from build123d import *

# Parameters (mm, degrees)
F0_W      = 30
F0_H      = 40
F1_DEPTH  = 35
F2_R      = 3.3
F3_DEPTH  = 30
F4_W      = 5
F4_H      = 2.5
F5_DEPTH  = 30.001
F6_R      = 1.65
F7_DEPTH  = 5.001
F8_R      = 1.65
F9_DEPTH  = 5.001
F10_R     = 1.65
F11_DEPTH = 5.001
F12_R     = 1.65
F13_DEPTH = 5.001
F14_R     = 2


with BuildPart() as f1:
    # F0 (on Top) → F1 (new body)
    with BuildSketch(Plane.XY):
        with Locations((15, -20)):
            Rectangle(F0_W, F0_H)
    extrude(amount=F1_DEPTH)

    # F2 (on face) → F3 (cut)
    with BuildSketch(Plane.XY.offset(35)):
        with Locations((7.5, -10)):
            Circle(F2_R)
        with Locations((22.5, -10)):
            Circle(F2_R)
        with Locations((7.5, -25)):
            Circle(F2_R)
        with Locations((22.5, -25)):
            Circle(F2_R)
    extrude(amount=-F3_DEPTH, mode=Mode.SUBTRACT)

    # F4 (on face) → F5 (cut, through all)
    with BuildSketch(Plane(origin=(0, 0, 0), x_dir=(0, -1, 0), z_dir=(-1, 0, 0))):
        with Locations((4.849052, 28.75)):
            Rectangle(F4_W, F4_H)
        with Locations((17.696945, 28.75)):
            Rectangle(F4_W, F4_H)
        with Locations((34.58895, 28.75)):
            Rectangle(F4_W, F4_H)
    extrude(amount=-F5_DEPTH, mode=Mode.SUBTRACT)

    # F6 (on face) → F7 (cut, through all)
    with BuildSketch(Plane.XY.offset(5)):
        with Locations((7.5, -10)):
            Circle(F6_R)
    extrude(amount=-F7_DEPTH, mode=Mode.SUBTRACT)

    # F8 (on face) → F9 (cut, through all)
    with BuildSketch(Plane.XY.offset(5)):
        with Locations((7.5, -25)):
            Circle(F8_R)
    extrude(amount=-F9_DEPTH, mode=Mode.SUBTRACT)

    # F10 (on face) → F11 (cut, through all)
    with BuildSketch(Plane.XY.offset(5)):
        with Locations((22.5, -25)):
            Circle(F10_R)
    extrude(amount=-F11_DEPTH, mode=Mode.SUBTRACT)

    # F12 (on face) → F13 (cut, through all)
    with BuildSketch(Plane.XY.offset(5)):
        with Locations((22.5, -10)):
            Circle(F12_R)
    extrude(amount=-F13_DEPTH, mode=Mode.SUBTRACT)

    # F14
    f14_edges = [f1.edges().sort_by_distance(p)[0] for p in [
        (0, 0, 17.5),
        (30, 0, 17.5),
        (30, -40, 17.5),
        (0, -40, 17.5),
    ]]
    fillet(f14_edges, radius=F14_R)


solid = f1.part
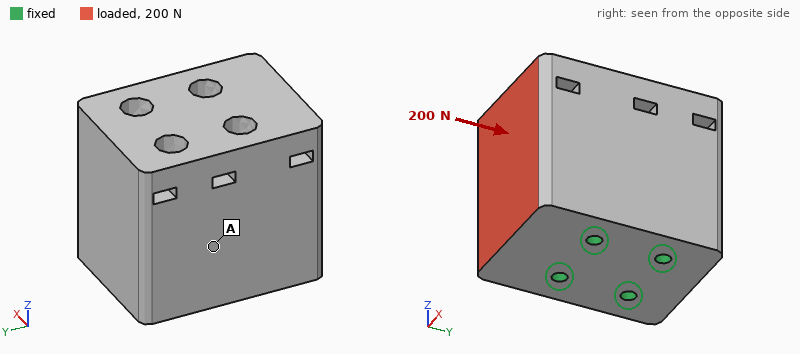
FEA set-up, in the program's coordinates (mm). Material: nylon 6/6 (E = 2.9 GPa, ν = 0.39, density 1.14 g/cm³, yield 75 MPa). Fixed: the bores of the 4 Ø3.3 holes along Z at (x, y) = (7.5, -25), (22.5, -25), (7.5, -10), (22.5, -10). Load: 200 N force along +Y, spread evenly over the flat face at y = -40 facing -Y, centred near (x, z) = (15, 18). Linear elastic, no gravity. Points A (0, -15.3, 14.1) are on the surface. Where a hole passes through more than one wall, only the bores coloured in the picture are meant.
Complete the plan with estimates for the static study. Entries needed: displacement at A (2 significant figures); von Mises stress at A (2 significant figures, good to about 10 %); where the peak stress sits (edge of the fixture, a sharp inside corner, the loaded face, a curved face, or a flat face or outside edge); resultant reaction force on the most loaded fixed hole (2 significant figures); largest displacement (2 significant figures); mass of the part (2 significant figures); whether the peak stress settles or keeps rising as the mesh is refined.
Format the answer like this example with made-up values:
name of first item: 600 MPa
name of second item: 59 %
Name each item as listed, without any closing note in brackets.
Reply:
displacement at A: 9.9 µm
von Mises stress at A: 0.52 MPa
where the peak stress sits: edge of the fixture
resultant reaction force on the most loaded fixed hole: 100 N
largest displacement: 33 µm
mass of the part: 42 g
whether the peak stress settles or keeps rising as the mesh is refined: keeps rising
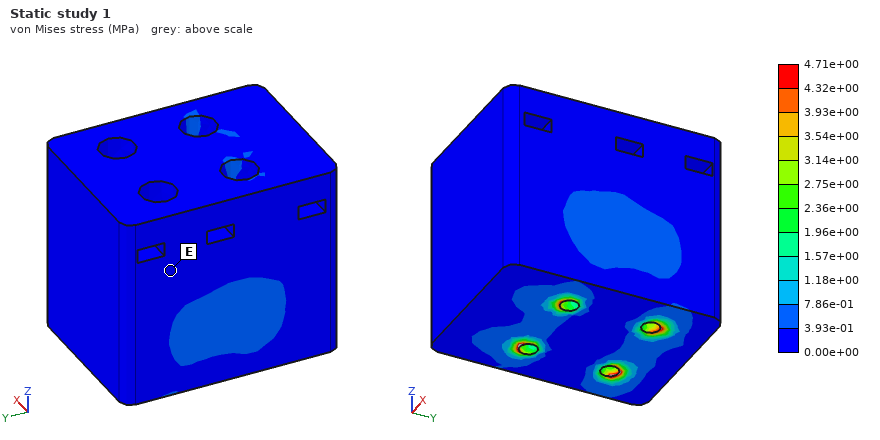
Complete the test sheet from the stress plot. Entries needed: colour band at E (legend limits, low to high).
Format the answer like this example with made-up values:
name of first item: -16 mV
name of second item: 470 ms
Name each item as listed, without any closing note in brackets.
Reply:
colour band at E: 0.00e+00 to 3.93e-01 MPa
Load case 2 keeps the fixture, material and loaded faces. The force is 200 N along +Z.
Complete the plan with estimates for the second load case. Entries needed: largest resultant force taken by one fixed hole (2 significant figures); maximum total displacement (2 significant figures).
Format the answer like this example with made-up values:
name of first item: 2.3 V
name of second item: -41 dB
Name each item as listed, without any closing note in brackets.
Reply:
largest resultant force taken by one fixed hole: 170 N
maximum total displacement: 47 µm
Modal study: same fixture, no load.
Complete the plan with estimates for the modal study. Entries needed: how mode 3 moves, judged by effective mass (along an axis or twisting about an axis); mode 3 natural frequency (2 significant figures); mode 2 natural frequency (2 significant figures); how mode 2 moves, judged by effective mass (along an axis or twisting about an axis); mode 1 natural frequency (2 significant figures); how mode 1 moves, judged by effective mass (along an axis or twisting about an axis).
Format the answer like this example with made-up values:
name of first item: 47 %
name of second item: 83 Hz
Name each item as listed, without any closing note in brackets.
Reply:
how mode 3 moves, judged by effective mass: twisting about Z
mode 3 natural frequency: 4800 Hz
mode 2 natural frequency: 2500 Hz
how mode 2 moves, judged by effective mass: along X
mode 1 natural frequency: 2300 Hz
how mode 1 moves, judged by effective mass: along Y
